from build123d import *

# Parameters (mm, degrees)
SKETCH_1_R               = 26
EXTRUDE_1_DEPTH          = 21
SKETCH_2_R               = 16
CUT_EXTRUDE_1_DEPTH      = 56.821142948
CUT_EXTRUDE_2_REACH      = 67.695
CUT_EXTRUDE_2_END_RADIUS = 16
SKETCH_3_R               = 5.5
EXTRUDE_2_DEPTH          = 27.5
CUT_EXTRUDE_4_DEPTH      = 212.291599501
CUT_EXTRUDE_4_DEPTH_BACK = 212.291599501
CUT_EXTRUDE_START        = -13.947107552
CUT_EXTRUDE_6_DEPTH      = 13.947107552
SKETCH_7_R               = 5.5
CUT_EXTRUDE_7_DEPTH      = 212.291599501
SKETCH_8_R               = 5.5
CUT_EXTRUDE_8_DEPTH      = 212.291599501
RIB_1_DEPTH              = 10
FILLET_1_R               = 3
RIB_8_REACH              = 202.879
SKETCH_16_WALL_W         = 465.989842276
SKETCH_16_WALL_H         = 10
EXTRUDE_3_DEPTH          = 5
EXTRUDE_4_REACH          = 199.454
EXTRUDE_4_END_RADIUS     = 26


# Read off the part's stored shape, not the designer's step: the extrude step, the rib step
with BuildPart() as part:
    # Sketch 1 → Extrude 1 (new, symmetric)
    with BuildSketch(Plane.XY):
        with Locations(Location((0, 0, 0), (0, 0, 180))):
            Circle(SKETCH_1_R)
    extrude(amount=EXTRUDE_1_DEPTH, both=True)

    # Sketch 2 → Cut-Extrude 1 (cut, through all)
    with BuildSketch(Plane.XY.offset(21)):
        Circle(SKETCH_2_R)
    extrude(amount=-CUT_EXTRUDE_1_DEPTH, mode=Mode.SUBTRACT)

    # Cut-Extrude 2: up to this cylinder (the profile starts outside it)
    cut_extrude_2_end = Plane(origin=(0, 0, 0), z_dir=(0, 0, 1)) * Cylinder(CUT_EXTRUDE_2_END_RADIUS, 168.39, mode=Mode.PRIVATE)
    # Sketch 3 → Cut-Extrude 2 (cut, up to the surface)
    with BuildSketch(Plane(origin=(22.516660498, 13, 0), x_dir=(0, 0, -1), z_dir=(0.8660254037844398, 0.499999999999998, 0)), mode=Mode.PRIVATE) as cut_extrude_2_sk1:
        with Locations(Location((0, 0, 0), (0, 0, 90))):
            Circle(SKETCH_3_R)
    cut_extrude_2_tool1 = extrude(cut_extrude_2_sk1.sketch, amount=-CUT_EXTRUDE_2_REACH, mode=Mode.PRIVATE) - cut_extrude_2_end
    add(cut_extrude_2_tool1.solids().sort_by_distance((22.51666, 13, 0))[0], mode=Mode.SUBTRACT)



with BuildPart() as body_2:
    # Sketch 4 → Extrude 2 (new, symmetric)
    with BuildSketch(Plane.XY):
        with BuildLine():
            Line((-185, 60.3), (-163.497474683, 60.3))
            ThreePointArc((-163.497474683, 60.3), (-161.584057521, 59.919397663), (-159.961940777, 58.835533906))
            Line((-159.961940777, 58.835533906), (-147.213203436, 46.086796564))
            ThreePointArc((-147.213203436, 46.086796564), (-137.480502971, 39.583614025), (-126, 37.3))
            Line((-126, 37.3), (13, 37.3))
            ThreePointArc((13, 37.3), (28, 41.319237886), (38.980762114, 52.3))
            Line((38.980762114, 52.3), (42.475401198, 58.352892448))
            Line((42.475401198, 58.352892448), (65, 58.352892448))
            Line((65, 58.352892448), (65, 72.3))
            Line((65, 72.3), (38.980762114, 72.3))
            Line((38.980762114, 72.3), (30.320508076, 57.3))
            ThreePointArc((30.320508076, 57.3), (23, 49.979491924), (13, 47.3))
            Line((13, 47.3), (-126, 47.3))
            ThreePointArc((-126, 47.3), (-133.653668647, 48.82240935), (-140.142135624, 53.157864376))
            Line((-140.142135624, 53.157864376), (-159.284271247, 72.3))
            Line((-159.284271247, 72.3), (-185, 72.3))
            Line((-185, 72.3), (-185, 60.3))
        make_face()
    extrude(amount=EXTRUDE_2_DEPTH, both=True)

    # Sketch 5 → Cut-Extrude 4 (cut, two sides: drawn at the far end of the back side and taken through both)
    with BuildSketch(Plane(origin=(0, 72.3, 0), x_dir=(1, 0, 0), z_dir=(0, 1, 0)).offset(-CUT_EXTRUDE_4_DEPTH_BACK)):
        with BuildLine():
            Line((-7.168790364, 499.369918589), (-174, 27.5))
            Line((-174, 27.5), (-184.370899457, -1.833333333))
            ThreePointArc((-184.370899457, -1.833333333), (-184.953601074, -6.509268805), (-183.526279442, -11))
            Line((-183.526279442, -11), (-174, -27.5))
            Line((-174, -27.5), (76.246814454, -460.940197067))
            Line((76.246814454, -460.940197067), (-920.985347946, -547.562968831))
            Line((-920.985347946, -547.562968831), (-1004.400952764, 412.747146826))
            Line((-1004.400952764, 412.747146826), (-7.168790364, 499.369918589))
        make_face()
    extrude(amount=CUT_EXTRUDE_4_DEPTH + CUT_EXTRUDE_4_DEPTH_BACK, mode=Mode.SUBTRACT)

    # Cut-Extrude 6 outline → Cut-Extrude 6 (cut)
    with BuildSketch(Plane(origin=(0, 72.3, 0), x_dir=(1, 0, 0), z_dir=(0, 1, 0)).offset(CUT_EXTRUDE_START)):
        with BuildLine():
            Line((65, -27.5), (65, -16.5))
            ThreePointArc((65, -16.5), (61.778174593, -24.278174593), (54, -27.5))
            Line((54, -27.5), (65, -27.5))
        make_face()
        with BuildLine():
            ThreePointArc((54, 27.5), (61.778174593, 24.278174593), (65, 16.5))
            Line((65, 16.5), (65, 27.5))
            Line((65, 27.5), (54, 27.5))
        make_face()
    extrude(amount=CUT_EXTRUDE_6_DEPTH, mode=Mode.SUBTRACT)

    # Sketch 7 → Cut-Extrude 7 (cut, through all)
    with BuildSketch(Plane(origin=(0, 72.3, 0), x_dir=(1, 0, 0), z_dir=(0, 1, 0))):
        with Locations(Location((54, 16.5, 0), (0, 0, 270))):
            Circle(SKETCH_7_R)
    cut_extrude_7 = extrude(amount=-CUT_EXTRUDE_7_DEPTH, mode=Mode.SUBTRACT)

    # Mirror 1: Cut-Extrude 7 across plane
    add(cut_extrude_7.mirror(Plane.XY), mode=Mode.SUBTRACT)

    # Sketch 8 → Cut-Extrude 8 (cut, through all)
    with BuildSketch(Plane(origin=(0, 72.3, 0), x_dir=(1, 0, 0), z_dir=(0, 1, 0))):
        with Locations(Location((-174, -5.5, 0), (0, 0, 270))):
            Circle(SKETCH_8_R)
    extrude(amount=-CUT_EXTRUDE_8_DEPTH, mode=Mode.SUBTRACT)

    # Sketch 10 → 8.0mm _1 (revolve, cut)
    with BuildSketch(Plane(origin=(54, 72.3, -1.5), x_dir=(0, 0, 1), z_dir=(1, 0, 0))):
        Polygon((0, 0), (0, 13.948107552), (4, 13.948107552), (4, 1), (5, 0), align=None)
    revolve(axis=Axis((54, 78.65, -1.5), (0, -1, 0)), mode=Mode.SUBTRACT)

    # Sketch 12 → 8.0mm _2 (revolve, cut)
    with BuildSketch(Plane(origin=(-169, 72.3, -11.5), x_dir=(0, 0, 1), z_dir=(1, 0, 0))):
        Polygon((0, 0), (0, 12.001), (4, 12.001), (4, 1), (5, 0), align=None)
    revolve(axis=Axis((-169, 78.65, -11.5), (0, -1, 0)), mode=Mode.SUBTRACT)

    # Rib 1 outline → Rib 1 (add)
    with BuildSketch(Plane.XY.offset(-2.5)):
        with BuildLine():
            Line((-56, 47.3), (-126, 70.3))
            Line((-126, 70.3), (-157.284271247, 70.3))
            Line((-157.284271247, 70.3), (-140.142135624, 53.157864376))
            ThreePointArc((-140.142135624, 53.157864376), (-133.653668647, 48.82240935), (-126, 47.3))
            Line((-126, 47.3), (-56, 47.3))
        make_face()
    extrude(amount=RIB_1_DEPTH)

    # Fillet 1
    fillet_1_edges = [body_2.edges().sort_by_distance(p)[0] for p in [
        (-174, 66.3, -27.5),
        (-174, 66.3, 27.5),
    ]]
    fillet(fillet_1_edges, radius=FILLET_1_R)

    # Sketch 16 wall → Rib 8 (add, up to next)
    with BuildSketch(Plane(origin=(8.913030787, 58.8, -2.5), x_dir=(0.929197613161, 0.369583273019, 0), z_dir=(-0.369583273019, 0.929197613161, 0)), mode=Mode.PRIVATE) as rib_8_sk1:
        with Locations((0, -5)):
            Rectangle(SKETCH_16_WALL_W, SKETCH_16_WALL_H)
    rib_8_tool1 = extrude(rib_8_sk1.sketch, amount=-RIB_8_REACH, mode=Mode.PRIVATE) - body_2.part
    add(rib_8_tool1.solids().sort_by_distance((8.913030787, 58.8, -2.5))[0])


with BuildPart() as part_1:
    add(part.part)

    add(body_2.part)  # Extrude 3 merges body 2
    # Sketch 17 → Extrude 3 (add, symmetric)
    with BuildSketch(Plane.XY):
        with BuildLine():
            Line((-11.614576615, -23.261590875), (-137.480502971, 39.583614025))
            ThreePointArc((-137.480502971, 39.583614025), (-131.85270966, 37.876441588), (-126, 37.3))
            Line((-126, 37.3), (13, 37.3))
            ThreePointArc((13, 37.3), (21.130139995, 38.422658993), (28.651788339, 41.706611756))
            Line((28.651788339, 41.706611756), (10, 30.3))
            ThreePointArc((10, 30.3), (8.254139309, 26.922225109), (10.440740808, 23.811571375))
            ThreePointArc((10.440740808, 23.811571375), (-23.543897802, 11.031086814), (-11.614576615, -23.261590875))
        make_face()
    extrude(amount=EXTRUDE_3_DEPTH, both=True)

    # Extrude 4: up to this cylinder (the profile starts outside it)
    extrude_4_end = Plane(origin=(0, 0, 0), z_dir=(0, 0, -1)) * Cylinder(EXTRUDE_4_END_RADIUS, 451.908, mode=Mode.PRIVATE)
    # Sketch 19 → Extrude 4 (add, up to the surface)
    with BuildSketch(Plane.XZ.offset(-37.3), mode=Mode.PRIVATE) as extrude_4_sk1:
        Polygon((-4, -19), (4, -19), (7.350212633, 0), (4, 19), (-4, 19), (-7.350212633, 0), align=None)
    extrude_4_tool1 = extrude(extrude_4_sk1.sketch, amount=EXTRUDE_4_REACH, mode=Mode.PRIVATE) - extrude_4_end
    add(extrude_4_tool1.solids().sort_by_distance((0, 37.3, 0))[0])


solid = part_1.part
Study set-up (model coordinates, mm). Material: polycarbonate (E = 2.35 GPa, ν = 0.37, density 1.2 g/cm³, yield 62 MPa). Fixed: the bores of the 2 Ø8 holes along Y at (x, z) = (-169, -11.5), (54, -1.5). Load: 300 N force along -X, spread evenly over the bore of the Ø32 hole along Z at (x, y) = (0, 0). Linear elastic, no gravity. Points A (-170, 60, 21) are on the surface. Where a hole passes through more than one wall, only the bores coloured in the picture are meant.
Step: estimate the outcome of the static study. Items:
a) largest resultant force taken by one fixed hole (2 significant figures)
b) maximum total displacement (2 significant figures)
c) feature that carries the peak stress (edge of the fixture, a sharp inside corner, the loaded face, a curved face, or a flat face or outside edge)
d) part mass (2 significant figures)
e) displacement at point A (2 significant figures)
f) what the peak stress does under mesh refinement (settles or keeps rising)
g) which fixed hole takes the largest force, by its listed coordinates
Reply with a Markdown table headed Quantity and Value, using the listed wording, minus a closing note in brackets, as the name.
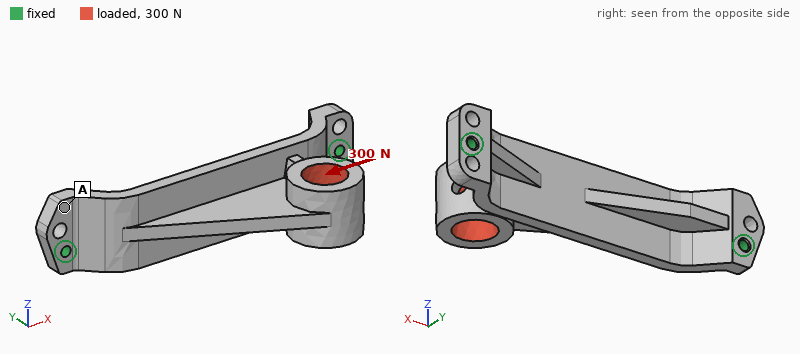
| Quantity | Value |
|---|---|
| largest resultant force taken by one fixed hole | 200 N |
| maximum total displacement | 96 µm |
| feature that carries the peak stress | edge of the fixture |
| part mass | 310 g |
| displacement at point A | 27 µm |
| what the peak stress does under mesh refinement | keeps rising |
| which fixed hole takes the largest force, by its listed coordinates | (-169, -11.5) |
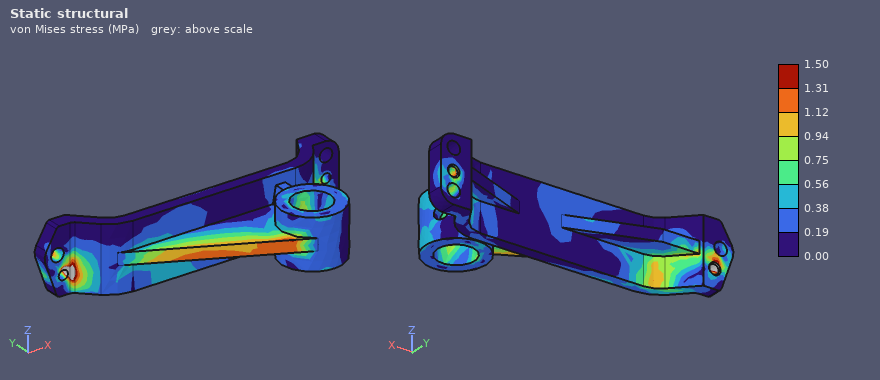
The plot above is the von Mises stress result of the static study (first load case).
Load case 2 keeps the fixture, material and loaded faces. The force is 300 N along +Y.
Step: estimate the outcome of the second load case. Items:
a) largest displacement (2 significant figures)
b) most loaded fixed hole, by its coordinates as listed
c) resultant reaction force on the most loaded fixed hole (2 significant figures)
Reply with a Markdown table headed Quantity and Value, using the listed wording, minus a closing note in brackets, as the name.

| Quantity | Value |
|---|---|
| largest displacement | 0.15 mm |
| most loaded fixed hole, by its coordinates as listed | (54, -1.5) |
| resultant reaction force on the most loaded fixed hole | 310 N |
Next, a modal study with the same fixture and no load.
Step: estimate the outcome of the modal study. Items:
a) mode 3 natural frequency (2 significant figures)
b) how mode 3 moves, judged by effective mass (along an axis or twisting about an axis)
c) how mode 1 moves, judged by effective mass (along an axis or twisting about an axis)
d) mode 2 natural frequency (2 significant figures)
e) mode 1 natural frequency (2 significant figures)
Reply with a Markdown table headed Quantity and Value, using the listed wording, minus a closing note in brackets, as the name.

| Quantity | Value |
|---|---|
| mode 3 natural frequency | 750 Hz |
| how mode 3 moves, judged by effective mass | along Y |
| how mode 1 moves, judged by effective mass | along Z |
| mode 2 natural frequency | 560 Hz |
| mode 1 natural frequency | 240 Hz |
